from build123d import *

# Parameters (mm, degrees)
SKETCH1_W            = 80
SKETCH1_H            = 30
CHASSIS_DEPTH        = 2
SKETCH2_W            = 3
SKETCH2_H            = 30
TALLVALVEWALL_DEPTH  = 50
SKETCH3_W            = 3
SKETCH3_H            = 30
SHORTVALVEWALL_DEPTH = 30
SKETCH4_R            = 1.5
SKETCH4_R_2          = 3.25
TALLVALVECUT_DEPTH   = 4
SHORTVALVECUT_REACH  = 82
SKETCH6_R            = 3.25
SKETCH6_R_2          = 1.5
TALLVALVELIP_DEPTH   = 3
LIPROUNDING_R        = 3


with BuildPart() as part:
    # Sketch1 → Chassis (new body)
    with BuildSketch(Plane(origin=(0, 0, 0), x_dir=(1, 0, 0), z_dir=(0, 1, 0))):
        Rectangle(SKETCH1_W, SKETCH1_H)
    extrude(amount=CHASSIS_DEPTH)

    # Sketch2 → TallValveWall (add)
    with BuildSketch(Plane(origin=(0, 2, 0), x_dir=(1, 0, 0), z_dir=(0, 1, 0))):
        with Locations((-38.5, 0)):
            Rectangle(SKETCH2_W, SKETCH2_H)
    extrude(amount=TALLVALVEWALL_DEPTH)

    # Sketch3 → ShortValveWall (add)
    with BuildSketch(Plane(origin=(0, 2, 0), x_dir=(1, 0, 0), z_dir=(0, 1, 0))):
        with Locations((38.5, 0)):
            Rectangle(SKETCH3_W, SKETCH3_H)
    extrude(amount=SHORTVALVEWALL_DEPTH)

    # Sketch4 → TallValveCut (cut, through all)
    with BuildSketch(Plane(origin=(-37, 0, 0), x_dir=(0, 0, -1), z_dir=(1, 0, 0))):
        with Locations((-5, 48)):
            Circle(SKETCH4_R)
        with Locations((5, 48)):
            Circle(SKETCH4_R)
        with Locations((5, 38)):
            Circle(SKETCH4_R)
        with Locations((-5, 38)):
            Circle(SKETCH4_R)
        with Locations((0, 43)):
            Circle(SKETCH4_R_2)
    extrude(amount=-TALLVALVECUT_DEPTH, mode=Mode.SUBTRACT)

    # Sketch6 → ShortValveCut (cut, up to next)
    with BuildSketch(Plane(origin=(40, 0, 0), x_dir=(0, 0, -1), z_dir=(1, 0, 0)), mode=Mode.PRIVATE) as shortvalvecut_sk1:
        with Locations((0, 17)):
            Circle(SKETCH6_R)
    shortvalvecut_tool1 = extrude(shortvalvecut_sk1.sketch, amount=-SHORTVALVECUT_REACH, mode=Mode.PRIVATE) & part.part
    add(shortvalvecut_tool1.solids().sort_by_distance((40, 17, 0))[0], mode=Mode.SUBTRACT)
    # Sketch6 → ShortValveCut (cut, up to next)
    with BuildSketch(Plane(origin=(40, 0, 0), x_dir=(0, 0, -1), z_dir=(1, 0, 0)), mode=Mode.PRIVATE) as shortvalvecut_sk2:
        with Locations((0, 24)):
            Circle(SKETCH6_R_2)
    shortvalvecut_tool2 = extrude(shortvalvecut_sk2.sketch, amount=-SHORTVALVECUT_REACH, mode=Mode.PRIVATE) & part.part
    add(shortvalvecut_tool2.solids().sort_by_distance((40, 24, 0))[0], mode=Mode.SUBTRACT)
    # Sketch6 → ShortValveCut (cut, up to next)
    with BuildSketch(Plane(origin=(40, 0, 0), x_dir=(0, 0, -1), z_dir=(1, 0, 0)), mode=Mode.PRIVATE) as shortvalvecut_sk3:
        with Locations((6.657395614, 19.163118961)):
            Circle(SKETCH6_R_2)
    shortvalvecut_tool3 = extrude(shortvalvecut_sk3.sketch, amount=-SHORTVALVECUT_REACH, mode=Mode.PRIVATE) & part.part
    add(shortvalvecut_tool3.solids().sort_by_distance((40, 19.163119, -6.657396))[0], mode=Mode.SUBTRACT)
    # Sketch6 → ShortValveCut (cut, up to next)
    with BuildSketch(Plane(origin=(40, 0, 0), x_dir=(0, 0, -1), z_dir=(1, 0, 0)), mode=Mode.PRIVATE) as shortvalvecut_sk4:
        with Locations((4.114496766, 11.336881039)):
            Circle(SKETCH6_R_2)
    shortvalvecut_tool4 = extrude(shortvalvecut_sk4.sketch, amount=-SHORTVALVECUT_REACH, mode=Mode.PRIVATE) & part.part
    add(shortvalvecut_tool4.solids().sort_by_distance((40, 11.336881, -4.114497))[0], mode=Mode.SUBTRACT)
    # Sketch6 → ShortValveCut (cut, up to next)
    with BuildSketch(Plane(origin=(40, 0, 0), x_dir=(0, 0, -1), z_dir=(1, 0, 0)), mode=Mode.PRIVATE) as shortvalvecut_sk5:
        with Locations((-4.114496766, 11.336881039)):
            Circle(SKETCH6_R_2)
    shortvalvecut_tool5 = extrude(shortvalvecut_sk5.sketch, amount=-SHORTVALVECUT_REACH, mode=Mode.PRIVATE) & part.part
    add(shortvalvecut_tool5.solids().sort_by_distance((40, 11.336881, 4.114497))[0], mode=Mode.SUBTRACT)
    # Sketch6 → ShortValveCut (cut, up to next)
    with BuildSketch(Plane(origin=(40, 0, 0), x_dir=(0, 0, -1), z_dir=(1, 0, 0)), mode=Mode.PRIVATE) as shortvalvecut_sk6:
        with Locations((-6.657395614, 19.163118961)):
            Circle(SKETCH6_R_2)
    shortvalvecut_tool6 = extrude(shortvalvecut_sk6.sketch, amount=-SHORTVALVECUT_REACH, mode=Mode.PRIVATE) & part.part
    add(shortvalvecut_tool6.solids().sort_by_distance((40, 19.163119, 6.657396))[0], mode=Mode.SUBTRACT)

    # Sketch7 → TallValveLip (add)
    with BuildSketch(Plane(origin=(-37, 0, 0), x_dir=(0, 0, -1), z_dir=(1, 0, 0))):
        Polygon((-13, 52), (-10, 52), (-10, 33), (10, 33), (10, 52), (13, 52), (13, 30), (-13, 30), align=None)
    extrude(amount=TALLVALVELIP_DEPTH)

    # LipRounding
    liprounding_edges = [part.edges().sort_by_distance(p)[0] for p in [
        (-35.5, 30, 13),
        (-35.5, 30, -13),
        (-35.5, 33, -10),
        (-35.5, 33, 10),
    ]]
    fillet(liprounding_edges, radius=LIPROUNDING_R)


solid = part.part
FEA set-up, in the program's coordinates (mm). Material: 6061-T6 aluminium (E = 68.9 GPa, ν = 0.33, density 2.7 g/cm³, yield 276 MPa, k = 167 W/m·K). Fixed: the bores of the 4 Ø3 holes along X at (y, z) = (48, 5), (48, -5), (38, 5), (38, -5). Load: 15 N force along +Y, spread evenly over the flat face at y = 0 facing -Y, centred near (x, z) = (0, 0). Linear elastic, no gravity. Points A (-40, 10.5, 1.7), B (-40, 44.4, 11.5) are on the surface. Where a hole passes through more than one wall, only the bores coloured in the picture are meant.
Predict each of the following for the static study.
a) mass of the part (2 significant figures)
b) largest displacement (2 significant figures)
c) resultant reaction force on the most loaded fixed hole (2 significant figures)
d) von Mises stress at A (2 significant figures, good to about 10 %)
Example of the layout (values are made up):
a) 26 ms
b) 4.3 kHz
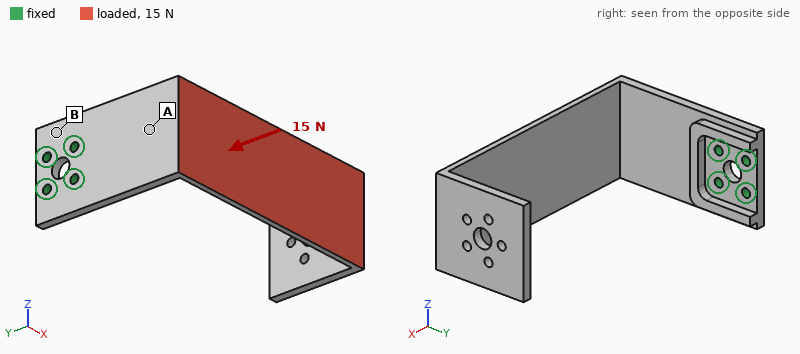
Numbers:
a) 33 g
b) 0.96 mm
c) 17 N
d) 11 MPa
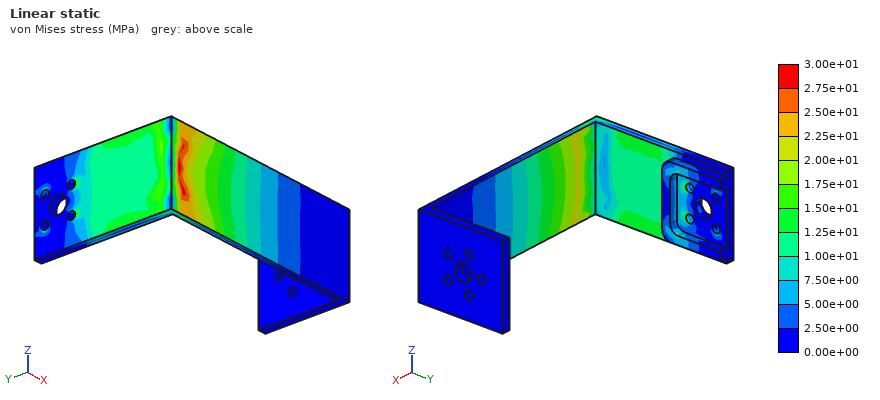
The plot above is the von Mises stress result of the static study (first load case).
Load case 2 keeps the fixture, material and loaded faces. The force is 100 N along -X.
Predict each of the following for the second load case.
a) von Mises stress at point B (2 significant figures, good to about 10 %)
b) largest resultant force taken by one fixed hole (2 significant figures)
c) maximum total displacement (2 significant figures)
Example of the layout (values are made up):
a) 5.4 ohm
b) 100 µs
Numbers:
a) 7.5 MPa
b) 150 N
c) 1.2 mm
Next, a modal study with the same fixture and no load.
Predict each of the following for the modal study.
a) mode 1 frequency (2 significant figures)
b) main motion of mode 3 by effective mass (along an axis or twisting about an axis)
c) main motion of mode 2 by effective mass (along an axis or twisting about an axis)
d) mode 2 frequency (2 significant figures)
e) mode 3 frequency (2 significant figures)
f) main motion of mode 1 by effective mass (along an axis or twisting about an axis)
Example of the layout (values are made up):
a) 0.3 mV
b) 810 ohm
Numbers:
a) 130 Hz
b) along X
c) along Z
d) 270 Hz
e) 530 Hz
f) along Y
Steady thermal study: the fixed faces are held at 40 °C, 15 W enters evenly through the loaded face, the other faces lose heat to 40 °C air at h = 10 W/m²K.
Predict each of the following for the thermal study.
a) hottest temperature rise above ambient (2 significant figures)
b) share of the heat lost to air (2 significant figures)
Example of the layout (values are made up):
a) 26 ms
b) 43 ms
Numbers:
a) 69 K
b) 22 %
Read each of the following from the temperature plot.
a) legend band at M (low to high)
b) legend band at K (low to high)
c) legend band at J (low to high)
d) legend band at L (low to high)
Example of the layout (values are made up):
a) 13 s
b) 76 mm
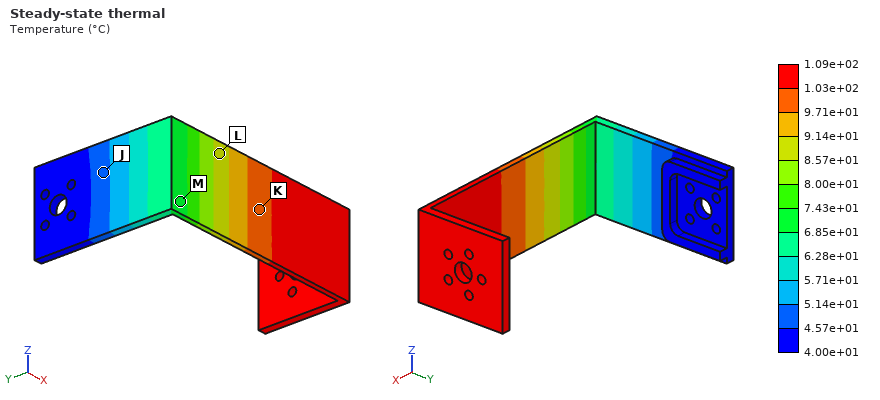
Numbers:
a) 6.85e+01 to 7.43e+01 °C
b) 9.71e+01 to 1.03e+02 °C
c) 4.57e+01 to 5.14e+01 °C
d) 8.57e+01 to 9.14e+01 °C
